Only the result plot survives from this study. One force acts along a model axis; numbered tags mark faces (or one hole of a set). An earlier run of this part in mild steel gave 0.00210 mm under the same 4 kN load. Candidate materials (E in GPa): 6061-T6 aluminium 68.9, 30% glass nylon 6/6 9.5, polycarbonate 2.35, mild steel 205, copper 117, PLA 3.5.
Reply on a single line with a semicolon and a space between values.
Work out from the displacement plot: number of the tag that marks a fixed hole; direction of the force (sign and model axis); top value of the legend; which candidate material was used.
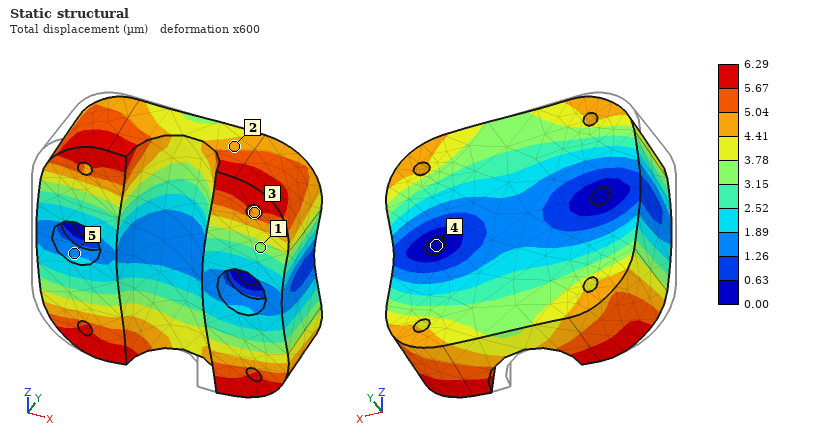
4; +X; 6.29 µm; 6061-T6 aluminium
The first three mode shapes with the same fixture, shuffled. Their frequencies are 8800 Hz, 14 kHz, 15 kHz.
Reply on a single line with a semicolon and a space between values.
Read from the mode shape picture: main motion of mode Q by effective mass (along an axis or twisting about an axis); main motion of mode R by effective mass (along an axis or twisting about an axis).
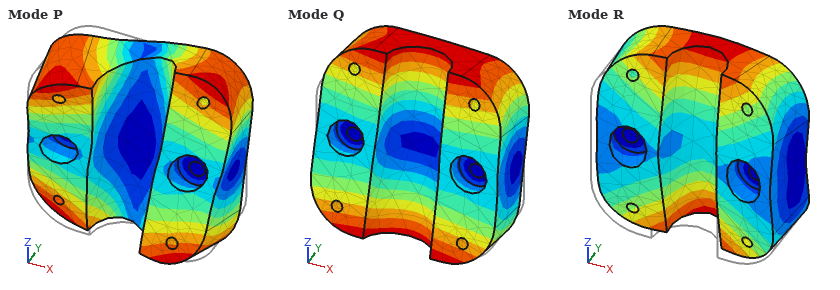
twisting about X; along Y
